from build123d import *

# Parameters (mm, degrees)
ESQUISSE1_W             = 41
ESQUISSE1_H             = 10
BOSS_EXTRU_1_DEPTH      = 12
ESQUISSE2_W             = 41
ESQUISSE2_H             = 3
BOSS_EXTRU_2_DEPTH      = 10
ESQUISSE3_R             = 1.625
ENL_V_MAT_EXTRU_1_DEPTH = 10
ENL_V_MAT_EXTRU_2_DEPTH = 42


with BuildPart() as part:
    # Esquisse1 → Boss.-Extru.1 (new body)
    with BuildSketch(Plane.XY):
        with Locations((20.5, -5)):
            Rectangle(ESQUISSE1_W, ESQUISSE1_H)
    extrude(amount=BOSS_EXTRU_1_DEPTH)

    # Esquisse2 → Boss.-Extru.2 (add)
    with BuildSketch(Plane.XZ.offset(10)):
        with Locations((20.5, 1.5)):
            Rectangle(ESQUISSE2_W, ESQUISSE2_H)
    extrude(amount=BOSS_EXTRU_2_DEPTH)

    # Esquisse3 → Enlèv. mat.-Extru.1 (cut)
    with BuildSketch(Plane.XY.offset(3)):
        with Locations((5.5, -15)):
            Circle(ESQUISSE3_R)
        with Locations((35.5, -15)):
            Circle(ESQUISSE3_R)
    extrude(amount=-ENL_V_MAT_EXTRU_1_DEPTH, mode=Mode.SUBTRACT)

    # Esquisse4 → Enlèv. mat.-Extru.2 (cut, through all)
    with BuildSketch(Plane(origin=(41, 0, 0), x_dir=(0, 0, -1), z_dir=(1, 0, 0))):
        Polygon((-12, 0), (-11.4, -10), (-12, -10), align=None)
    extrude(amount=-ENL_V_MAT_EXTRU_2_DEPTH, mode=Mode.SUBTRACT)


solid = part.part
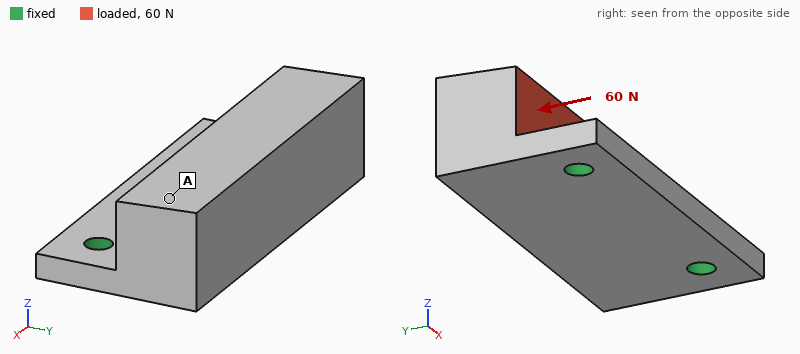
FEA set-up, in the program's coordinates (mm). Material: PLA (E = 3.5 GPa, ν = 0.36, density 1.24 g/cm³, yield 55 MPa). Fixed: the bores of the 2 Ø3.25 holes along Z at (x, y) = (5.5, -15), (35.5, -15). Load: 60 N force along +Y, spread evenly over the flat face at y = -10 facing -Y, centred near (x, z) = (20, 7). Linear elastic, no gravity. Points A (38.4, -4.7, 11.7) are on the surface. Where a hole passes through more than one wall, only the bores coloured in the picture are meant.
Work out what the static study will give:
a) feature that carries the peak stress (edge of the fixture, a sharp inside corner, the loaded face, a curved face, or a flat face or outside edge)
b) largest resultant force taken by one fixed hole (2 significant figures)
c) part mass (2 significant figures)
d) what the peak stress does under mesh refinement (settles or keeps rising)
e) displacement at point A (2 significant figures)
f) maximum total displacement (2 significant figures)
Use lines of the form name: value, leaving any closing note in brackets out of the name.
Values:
feature that carries the peak stress: edge of the fixture
largest resultant force taken by one fixed hole: 31 N
part mass: 7.4 g
what the peak stress does under mesh refinement: keeps rising
displacement at point A: 0.100 mm
maximum total displacement: 0.13 mm
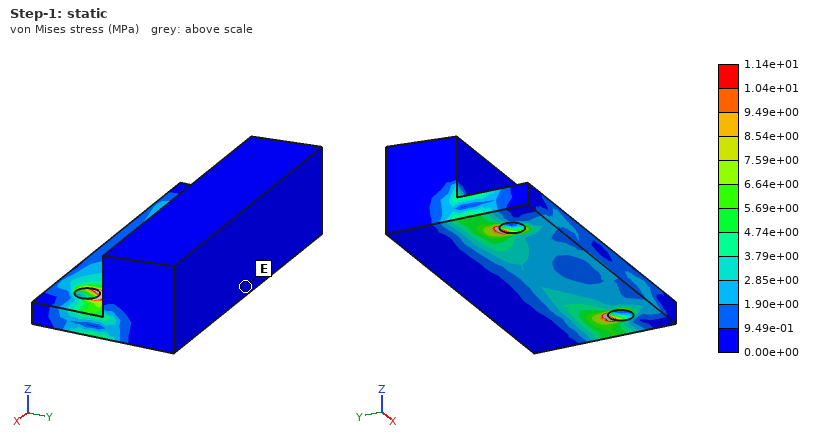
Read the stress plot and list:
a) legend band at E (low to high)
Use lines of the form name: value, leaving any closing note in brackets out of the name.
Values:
legend band at E: 0.00e+00 to 9.49e-01 MPa
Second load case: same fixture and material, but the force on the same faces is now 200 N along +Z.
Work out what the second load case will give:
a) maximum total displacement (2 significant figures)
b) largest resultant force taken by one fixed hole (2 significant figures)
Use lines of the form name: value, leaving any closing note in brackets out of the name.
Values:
maximum total displacement: 0.17 mm
largest resultant force taken by one fixed hole: 100 N
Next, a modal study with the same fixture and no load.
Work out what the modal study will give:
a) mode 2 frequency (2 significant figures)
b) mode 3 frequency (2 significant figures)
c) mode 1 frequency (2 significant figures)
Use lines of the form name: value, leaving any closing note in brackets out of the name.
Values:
mode 2 frequency: 4300 Hz
mode 3 frequency: 6300 Hz
mode 1 frequency: 1400 Hz
